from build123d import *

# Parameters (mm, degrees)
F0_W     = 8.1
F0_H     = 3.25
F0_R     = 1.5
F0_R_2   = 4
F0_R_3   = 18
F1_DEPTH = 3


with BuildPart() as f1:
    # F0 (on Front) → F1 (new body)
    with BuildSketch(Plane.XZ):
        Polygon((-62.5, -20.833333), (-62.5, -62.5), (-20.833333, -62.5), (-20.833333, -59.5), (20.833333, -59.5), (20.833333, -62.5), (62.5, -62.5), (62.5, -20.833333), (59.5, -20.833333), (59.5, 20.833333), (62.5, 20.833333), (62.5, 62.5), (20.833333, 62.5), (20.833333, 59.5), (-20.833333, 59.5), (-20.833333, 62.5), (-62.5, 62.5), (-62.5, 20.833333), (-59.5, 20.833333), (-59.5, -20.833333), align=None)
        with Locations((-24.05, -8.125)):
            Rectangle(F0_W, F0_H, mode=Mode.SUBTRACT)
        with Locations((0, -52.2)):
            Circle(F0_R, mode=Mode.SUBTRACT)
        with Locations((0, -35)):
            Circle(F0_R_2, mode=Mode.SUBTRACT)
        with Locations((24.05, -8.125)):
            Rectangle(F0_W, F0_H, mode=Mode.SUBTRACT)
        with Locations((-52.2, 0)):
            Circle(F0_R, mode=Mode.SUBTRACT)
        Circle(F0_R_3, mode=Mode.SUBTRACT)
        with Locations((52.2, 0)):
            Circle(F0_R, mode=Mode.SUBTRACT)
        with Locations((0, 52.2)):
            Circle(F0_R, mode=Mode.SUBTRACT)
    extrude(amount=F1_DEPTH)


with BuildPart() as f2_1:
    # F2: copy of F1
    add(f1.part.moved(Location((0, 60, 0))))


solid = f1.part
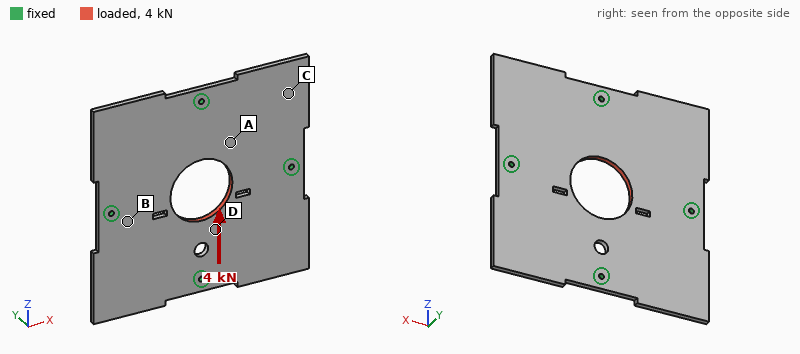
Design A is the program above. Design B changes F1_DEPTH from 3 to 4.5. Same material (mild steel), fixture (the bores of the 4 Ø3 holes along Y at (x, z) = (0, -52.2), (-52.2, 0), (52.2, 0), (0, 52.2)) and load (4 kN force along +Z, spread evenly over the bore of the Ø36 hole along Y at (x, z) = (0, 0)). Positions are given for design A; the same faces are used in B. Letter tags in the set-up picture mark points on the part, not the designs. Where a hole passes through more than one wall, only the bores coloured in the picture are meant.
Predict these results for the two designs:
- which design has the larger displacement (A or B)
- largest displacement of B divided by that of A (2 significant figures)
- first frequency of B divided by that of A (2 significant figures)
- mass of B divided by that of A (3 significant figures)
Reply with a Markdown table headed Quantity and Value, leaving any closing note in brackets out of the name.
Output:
| Quantity | Value |
|---|---|
| which design has the larger displacement | A |
| largest displacement of B divided by that of A | 0.66 |
| first frequency of B divided by that of A | 1.4 |
| mass of B divided by that of A | 1.50 |
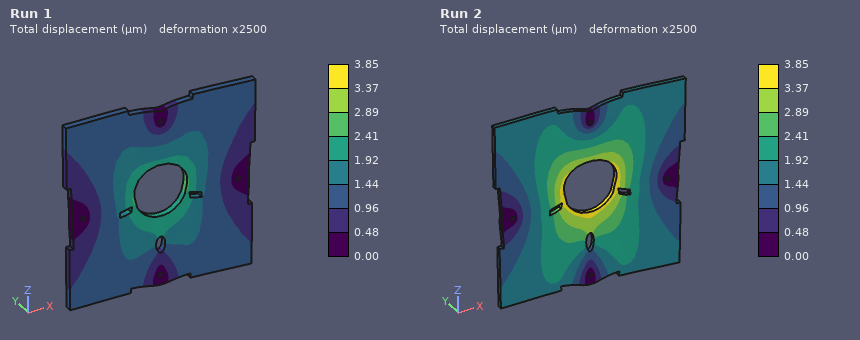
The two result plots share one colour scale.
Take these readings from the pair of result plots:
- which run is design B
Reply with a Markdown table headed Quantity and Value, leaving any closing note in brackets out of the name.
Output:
| Quantity | Value |
|---|---|
| which run is design B | Run 1 |
